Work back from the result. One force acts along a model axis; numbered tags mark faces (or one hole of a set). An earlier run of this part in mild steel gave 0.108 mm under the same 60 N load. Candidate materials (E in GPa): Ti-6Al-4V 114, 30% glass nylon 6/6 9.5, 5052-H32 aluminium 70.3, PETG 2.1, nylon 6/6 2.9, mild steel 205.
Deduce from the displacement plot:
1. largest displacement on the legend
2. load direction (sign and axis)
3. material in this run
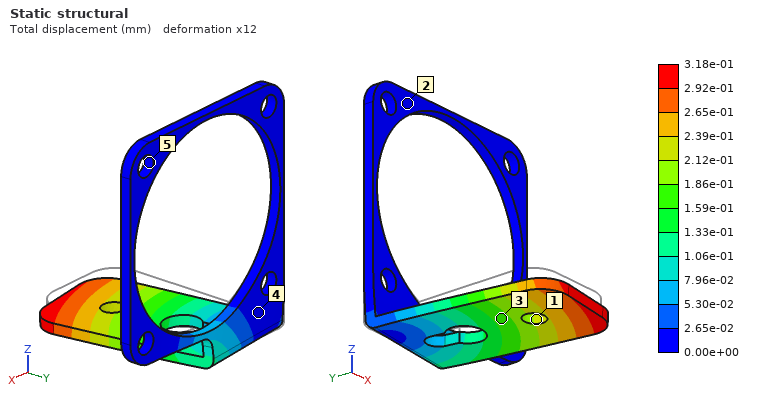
3.18e-01 mm
+X
5052-H32 aluminium
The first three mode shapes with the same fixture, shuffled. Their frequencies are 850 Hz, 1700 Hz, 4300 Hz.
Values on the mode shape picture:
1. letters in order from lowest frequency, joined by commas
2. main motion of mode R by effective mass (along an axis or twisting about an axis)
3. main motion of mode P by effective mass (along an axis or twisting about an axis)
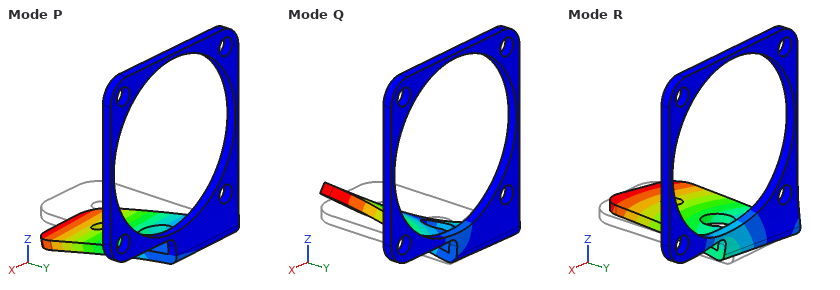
P, R, Q
along X
along Z
